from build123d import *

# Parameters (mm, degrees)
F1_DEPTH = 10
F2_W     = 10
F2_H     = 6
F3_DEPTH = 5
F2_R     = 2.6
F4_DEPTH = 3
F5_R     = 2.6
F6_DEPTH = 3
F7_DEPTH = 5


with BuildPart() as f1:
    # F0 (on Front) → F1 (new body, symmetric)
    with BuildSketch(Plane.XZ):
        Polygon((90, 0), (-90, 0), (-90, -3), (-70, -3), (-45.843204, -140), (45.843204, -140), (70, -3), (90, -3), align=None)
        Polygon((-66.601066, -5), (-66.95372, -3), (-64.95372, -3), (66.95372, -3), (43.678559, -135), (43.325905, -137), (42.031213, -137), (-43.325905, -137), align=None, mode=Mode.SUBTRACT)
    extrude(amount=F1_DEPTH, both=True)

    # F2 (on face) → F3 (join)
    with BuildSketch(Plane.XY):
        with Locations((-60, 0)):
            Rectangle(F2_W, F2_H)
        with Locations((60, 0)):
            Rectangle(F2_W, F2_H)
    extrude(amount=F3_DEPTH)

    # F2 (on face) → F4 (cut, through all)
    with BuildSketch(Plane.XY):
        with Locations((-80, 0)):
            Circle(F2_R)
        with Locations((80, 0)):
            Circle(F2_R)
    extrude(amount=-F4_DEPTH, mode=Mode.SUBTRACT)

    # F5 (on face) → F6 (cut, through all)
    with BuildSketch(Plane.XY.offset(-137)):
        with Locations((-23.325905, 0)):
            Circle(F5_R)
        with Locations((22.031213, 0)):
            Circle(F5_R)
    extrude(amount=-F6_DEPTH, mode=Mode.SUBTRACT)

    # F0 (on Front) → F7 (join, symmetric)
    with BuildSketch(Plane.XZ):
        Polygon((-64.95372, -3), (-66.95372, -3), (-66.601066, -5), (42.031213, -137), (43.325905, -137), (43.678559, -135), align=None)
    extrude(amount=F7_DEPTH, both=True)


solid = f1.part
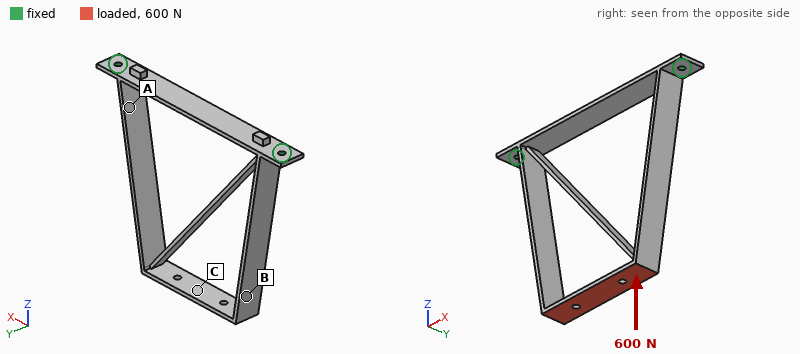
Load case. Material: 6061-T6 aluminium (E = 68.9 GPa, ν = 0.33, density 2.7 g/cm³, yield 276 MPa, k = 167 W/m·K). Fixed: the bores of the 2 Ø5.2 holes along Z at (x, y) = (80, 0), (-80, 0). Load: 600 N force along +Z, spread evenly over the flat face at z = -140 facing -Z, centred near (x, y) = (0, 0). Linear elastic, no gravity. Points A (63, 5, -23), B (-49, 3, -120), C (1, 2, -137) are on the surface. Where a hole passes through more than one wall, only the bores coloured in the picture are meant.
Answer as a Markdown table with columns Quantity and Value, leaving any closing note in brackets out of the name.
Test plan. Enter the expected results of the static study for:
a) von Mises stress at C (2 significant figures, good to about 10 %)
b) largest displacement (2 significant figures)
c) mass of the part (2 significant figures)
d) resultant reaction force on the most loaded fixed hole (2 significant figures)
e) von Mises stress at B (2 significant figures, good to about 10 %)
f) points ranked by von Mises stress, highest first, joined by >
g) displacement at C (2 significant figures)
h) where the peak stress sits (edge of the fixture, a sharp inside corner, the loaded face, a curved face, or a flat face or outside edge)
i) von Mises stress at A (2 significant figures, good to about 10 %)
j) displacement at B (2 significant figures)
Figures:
| Quantity | Value |
|---|---|
| von Mises stress at C | 120 MPa |
| largest displacement | 0.93 mm |
| mass of the part | 100 g |
| resultant reaction force on the most loaded fixed hole | 310 N |
| von Mises stress at B | 59 MPa |
| points ranked by von Mises stress, highest first, joined by > | C > B > A |
| displacement at C | 0.91 mm |
| where the peak stress sits | the loaded face |
| von Mises stress at A | 18 MPa |
| displacement at B | 0.37 mm |
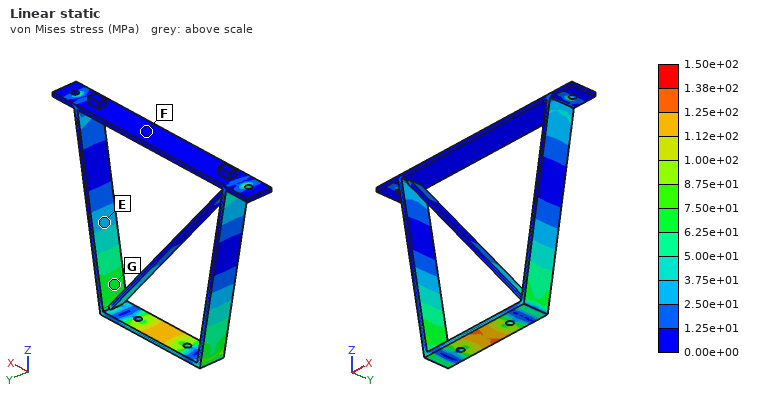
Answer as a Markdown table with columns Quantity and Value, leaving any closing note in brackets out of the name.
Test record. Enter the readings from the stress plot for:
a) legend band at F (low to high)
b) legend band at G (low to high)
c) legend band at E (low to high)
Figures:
| Quantity | Value |
|---|---|
| legend band at F | 0.00e+00 to 1.25e+01 MPa |
| legend band at G | 6.25e+01 to 7.50e+01 MPa |
| legend band at E | 2.50e+01 to 3.75e+01 MPa |
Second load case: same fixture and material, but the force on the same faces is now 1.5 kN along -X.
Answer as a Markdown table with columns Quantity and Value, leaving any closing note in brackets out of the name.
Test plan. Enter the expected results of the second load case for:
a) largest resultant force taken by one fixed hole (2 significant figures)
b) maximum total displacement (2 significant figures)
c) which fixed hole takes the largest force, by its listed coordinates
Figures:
| Quantity | Value |
|---|---|
| largest resultant force taken by one fixed hole | 1.8 kN |
| maximum total displacement | 0.57 mm |
| which fixed hole takes the largest force, by its listed coordinates | (-80, 0) |
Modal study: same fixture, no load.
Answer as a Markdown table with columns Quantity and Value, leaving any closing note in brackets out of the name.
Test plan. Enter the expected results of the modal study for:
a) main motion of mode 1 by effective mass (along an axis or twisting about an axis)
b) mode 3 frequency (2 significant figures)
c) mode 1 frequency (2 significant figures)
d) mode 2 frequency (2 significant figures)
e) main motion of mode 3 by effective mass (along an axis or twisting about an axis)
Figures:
| Quantity | Value |
|---|---|
| main motion of mode 1 by effective mass | along Y |
| mode 3 frequency | 480 Hz |
| mode 1 frequency | 210 Hz |
| mode 2 frequency | 410 Hz |
| main motion of mode 3 by effective mass | twisting about Z |
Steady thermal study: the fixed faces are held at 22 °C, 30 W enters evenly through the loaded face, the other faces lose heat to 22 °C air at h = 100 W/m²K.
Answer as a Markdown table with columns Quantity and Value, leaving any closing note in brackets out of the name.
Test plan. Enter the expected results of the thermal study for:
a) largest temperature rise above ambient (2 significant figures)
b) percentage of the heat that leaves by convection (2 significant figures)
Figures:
| Quantity | Value |
|---|---|
| largest temperature rise above ambient | 55 K |
| percentage of the heat that leaves by convection | 96 % |
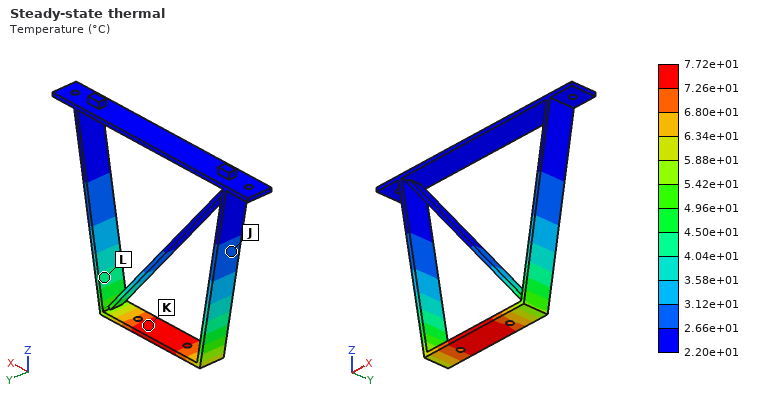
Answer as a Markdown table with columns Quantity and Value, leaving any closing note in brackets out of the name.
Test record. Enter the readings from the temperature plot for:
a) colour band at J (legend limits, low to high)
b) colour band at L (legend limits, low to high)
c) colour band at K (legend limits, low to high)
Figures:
| Quantity | Value |
|---|---|
| colour band at J | 2.66e+01 to 3.12e+01 °C |
| colour band at L | 4.04e+01 to 4.50e+01 °C |
| colour band at K | 7.26e+01 to 7.72e+01 °C |
